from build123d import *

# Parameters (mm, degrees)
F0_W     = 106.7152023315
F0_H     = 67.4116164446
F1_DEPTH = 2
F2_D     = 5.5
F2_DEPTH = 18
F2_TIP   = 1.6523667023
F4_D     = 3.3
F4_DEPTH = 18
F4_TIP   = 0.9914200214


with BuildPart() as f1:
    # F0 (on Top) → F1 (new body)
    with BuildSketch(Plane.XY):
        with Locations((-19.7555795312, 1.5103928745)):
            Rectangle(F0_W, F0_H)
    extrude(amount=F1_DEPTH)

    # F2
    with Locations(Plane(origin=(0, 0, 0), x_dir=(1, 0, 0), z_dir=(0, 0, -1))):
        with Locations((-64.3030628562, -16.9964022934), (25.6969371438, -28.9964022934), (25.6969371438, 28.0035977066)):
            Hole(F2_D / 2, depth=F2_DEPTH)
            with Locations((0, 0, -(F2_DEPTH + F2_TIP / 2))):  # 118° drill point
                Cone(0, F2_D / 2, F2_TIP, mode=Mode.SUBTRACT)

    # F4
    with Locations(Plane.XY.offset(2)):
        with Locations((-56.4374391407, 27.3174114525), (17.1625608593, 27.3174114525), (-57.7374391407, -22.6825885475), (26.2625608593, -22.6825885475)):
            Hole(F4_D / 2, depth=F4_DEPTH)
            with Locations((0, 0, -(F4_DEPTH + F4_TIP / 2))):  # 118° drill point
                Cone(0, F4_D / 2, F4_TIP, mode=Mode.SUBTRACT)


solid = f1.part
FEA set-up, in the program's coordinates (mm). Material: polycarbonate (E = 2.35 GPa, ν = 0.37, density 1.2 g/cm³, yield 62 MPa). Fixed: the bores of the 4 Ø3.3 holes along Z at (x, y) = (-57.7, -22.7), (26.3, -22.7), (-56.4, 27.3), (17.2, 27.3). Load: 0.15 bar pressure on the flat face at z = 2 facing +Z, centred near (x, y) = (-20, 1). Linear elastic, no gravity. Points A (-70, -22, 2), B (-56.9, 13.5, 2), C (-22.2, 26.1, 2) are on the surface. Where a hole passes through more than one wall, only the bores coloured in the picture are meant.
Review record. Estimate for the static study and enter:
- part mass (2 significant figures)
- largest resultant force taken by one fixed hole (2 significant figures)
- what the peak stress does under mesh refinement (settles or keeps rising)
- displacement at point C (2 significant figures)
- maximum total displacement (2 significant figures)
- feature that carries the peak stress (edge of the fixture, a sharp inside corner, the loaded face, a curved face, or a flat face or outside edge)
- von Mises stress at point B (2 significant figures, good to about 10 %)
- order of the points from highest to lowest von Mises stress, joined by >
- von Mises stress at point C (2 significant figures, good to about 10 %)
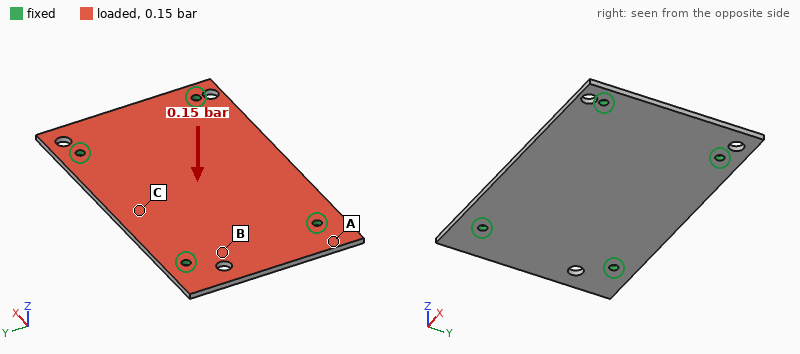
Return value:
17 g
30 N
keeps rising
0.90 mm
1.5 mm
edge of the fixture
4.1 MPa
C > B > A
5.6 MPa
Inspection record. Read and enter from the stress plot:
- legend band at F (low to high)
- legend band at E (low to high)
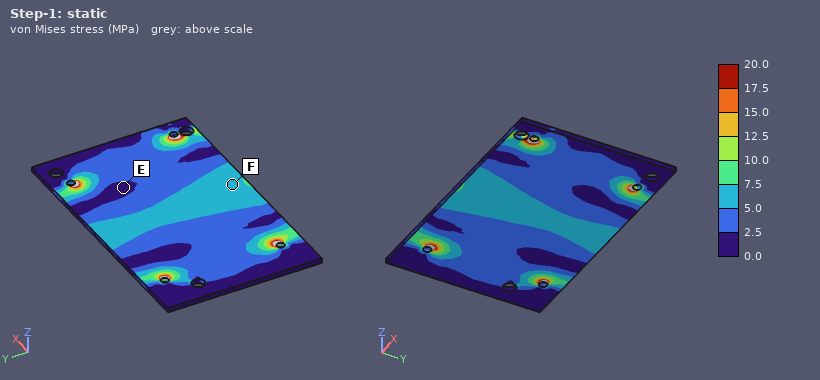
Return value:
5.0 to 7.5 MPa
0.0 to 2.5 MPa
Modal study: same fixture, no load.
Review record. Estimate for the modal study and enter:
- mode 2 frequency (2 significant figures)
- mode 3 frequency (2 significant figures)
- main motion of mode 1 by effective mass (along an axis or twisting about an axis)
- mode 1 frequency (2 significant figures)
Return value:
600 Hz
920 Hz
along Z
400 Hz
